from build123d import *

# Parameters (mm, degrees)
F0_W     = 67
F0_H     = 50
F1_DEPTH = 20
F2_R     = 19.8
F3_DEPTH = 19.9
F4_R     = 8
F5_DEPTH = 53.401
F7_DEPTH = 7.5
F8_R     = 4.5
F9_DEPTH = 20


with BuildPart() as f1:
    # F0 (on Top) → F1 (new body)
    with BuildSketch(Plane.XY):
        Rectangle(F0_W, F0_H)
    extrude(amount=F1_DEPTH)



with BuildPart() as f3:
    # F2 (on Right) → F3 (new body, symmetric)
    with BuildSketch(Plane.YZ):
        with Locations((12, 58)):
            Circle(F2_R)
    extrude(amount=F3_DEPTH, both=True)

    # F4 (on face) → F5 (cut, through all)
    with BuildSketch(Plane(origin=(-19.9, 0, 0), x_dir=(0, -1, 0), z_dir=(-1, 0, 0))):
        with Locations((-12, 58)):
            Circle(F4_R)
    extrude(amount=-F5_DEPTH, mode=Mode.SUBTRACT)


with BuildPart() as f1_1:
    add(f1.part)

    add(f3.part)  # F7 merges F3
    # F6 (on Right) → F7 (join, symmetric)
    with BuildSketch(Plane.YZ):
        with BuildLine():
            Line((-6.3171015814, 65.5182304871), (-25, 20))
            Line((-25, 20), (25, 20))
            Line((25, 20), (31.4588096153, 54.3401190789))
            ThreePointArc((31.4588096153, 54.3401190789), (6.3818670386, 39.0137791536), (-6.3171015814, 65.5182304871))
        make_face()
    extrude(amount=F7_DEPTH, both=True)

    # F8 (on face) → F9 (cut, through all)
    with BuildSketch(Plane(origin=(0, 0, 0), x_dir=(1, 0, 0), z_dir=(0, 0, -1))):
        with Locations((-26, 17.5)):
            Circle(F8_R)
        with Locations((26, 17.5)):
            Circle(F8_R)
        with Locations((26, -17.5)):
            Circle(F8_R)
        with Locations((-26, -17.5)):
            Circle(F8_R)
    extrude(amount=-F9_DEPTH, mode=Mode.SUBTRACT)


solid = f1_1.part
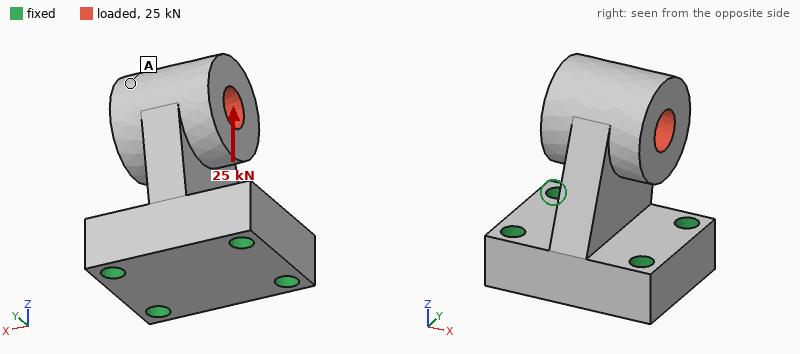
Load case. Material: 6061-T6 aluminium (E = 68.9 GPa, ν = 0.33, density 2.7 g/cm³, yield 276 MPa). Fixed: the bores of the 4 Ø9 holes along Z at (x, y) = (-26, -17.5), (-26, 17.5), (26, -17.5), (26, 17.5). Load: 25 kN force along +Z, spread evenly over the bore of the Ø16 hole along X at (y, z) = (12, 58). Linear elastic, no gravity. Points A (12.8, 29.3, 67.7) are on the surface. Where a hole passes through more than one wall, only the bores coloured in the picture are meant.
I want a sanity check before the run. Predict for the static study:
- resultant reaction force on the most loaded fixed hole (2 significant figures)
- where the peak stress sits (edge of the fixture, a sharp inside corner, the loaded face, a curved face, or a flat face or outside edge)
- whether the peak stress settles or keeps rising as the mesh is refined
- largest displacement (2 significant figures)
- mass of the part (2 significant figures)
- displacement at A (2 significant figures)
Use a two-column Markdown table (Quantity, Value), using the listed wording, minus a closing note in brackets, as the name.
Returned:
| Quantity | Value |
|---|---|
| resultant reaction force on the most loaded fixed hole | 10 kN |
| where the peak stress sits | edge of the fixture |
| whether the peak stress settles or keeps rising as the mesh is refined | keeps rising |
| largest displacement | 97 µm |
| mass of the part | 320 g |
| displacement at A | 95 µm |
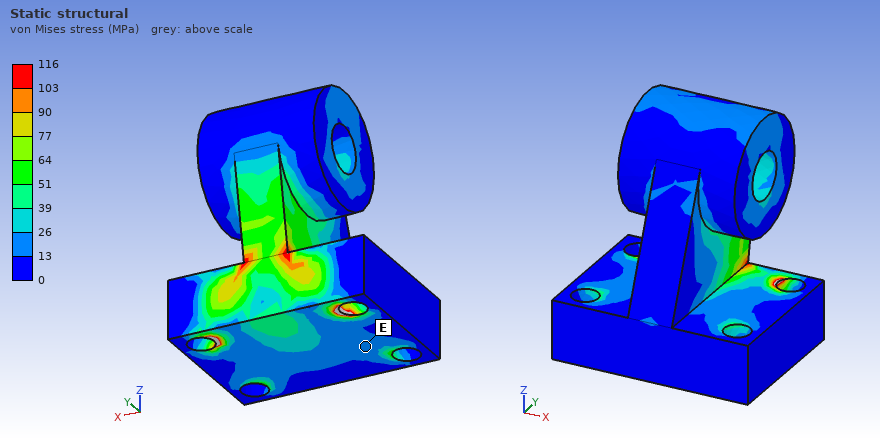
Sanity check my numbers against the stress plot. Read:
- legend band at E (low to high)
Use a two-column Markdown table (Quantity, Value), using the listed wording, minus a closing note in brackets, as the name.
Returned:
| Quantity | Value |
|---|---|
| legend band at E | 13 to 26 MPa |
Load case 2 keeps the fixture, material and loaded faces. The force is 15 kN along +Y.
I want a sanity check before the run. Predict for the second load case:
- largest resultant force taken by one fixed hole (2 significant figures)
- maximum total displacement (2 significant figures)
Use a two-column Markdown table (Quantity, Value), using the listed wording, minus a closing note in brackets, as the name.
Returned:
| Quantity | Value |
|---|---|
| largest resultant force taken by one fixed hole | 10 kN |
| maximum total displacement | 0.21 mm |
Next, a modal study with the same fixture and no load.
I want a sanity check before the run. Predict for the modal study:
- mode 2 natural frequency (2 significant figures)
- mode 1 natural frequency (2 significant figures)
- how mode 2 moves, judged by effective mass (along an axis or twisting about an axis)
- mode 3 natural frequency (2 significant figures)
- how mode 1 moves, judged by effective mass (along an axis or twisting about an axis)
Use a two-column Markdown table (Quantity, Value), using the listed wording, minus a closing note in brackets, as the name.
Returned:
| Quantity | Value |
|---|---|
| mode 2 natural frequency | 4300 Hz |
| mode 1 natural frequency | 2400 Hz |
| how mode 2 moves, judged by effective mass | along Y |
| mode 3 natural frequency | 6600 Hz |
| how mode 1 moves, judged by effective mass | along X |
